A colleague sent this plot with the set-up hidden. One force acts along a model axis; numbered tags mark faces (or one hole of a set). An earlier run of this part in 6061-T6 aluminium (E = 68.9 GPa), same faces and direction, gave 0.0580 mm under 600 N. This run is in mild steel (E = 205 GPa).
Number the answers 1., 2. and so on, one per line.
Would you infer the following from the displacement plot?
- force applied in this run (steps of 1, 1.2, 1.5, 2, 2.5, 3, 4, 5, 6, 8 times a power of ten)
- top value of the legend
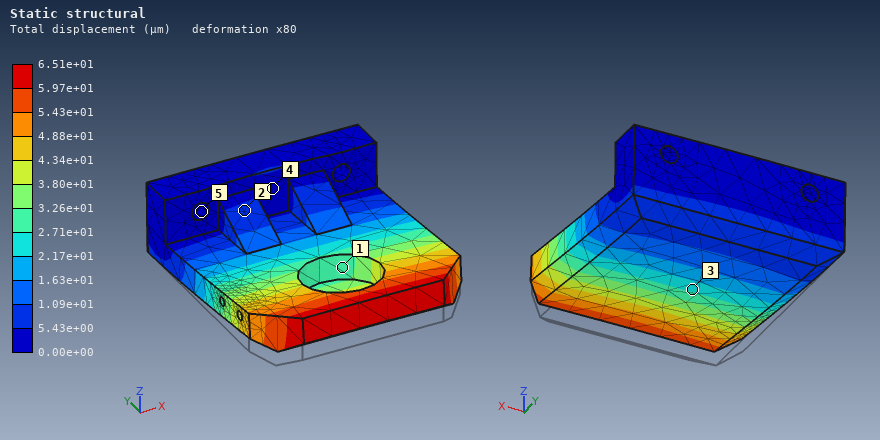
1. 2 kN
2. 6.51e+01 µm
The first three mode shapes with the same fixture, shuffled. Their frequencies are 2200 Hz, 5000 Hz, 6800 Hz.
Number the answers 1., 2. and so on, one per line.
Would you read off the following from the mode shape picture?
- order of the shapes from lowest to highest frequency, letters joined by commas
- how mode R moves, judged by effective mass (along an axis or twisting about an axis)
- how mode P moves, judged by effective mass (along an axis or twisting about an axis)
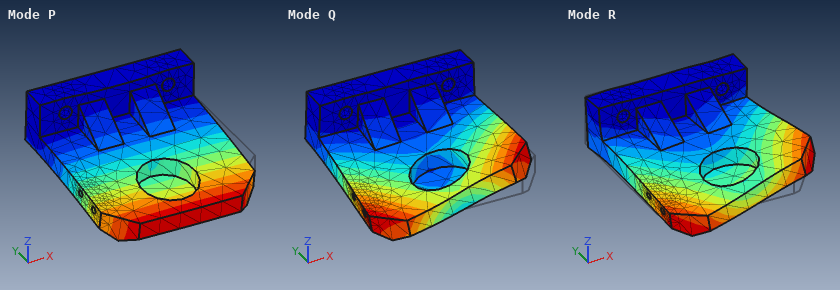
1. P, Q, R
2. along X
3. along Z
